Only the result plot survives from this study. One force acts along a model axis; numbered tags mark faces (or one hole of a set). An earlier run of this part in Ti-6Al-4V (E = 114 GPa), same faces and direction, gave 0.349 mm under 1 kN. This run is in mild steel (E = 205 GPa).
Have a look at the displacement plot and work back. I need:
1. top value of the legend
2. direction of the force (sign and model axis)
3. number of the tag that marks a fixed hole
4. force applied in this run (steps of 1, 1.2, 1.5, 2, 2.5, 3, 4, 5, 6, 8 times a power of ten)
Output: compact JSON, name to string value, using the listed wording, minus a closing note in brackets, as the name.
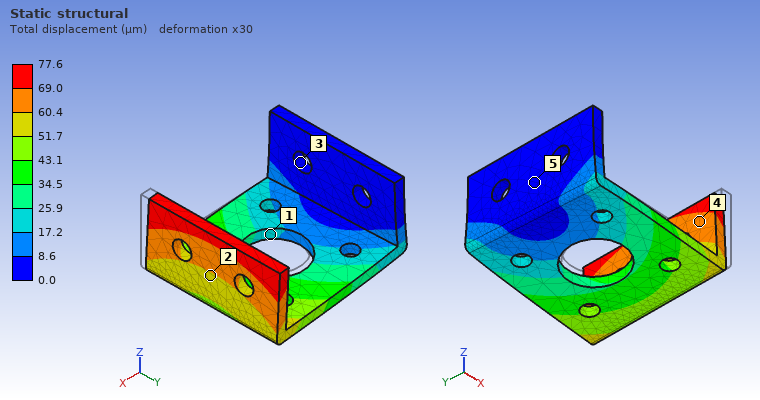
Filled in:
{"top value of the legend": "77.6 µm", "direction of the force": "+Y", "number of the tag that marks a fixed hole": "3", "force applied in this run": "400 N"}
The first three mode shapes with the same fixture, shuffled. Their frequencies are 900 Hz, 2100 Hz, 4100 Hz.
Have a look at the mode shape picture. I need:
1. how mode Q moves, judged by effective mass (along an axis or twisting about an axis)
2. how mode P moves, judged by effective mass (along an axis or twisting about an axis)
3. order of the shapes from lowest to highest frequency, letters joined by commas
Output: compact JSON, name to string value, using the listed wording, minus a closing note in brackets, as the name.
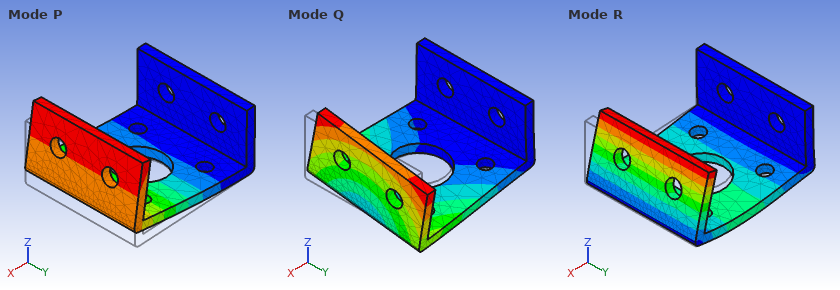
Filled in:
{"how mode Q moves, judged by effective mass": "along Y", "how mode P moves, judged by effective mass": "along Z", "order of the shapes from lowest to highest frequency, letters joined by commas": "P, Q, R"}
